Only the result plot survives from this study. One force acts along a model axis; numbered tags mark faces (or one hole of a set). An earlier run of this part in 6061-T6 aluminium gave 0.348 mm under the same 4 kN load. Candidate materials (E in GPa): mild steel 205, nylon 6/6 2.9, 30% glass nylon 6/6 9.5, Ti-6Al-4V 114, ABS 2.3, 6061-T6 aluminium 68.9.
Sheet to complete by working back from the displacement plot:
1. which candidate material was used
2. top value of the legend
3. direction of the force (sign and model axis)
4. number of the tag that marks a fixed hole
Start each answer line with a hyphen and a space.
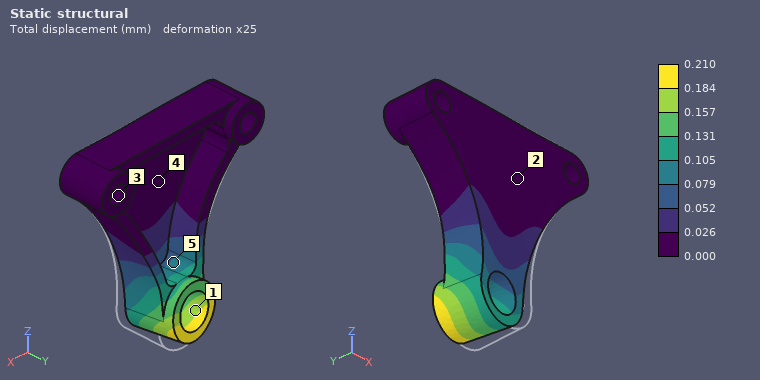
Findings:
- Ti-6Al-4V
- 0.210 mm
- -X
- 3
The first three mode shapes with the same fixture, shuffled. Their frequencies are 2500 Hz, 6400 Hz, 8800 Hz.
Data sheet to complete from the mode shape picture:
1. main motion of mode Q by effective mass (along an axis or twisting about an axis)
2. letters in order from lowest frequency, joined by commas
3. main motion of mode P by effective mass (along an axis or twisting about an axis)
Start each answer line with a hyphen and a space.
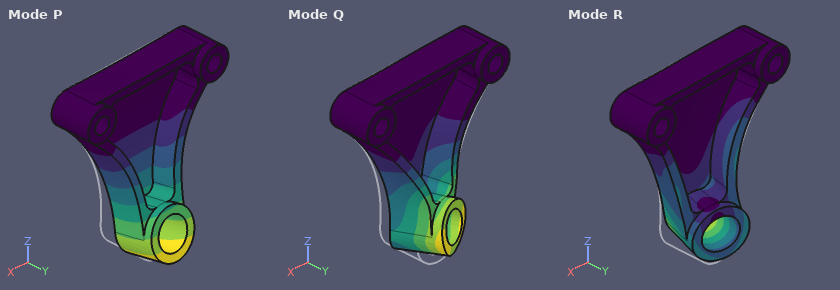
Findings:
- along X
- P, Q, R
- along Y
